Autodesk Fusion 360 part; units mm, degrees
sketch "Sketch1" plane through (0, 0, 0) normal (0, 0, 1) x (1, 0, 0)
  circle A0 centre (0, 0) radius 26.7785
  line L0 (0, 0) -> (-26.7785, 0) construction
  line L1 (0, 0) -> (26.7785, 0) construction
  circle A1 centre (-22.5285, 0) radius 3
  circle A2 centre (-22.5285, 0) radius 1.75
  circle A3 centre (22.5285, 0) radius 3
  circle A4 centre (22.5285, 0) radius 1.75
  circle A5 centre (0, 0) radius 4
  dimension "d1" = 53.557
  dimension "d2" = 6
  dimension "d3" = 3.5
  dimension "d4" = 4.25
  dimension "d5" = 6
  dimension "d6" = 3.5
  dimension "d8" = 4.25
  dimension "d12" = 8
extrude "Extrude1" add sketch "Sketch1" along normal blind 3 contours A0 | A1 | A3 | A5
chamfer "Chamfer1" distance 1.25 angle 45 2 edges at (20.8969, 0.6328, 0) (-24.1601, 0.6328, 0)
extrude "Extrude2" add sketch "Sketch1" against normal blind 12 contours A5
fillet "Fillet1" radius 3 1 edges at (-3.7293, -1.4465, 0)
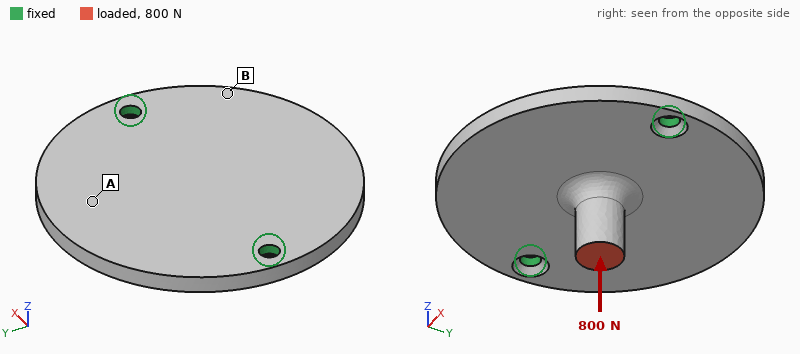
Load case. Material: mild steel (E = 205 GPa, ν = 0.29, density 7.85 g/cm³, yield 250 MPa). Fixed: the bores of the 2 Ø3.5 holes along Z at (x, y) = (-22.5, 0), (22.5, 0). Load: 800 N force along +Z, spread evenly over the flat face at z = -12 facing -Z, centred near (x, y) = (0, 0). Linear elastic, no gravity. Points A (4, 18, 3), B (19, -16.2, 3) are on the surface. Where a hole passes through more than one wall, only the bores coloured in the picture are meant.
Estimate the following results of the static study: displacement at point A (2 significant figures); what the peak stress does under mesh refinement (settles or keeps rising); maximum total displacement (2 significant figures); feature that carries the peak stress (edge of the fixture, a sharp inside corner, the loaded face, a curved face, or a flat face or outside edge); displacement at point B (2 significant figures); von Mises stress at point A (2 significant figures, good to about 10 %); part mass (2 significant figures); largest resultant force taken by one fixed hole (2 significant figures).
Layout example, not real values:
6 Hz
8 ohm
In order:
29 µm
keeps rising
32 µm
edge of the fixture
12 µm
32 MPa
58 g
560 N
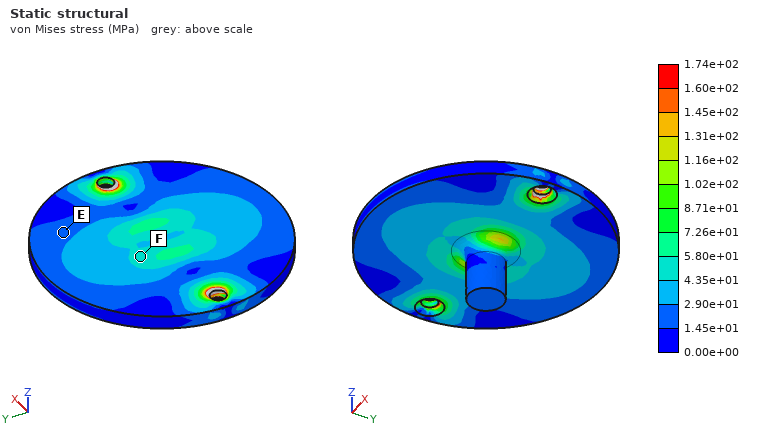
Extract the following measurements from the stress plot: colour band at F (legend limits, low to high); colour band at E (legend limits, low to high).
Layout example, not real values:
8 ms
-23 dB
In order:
4.35e+01 to 5.80e+01 MPa
1.45e+01 to 2.90e+01 MPa
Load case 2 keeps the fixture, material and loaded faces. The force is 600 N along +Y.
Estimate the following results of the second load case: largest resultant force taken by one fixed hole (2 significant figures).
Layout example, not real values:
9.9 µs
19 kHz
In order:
300 N
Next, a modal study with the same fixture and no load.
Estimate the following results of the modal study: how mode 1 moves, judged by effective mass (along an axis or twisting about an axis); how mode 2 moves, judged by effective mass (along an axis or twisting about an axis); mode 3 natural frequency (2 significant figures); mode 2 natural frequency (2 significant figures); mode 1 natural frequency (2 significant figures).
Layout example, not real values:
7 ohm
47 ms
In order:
twisting about X
along Z
8100 Hz
3600 Hz
2400 Hz
